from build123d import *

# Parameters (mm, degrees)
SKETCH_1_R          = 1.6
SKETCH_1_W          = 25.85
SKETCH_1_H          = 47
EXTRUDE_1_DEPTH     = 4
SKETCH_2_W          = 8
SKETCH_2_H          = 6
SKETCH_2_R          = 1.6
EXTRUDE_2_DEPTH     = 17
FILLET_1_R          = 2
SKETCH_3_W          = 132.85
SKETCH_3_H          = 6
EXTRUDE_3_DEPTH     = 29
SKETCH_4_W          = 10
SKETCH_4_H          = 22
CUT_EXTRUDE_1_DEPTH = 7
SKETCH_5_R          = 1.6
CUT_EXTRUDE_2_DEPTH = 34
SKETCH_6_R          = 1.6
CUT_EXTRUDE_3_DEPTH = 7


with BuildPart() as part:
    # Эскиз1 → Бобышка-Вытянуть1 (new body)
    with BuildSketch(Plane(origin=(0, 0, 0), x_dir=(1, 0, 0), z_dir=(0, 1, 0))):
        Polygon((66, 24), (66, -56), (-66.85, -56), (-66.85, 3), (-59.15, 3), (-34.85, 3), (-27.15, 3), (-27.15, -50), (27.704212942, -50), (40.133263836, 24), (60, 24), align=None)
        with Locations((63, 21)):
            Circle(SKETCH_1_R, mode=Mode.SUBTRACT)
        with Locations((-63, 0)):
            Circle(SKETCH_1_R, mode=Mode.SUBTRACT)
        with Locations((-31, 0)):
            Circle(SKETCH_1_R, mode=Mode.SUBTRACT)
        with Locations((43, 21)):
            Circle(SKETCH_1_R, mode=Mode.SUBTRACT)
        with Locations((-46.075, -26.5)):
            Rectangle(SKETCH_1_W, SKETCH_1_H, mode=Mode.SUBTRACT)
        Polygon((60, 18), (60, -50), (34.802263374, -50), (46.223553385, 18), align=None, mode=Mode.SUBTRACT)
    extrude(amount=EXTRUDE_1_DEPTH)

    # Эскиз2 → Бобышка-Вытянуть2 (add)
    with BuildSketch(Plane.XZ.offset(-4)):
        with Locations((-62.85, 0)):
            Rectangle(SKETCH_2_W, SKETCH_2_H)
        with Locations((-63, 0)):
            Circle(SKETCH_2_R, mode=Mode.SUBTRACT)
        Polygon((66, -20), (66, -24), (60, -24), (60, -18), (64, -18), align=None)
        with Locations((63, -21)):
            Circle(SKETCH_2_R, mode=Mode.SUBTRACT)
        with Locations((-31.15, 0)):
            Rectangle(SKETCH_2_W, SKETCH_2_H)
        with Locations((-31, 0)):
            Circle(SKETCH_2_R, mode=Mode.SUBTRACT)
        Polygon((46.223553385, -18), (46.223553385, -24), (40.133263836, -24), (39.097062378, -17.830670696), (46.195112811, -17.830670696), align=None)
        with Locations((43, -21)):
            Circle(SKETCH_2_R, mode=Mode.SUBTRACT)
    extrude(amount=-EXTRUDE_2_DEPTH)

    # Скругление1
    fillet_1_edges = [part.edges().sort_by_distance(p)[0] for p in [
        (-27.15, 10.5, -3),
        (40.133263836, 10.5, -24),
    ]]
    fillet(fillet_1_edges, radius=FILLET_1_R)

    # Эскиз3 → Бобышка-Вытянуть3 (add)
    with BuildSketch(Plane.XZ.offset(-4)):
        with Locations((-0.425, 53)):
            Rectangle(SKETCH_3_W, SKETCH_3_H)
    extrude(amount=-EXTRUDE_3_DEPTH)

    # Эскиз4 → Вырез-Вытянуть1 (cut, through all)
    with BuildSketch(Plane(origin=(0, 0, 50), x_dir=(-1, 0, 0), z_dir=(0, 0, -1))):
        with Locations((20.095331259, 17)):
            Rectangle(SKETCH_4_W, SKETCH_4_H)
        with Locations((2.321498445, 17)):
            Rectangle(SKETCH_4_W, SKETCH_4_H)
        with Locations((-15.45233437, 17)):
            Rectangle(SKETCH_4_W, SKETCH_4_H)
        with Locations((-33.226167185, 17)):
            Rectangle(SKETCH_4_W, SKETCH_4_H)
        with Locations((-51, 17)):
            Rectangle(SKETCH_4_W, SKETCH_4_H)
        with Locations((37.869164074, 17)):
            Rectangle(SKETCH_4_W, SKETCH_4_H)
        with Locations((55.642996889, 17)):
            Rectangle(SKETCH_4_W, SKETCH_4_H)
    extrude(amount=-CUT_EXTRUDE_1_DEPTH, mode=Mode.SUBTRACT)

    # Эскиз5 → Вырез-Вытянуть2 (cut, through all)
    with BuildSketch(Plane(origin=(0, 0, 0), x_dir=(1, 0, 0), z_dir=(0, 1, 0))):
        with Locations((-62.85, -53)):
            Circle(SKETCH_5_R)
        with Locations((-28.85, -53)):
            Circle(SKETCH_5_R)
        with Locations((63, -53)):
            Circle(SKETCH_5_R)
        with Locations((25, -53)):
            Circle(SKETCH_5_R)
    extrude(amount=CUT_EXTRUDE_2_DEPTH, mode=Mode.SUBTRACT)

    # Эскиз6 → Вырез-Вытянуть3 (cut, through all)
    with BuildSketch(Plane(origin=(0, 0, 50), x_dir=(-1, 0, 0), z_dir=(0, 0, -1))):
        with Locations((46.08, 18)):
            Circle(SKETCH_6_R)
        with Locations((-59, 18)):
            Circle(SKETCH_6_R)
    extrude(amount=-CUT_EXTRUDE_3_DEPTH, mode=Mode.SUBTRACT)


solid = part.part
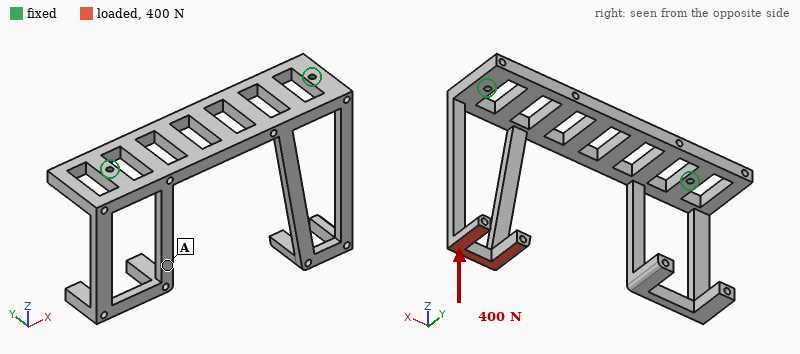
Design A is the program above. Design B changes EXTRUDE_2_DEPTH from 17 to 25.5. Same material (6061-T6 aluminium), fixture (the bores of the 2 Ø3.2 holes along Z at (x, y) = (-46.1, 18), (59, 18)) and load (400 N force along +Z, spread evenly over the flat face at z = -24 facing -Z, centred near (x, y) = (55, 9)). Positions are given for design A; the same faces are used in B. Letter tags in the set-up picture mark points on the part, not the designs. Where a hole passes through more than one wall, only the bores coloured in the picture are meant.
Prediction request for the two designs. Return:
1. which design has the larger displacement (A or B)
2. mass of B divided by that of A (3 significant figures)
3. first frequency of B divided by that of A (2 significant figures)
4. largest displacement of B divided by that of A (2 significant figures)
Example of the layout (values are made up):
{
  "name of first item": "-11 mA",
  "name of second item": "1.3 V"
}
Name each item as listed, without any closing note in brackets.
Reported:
{
  "which design has the larger displacement": "B",
  "mass of B divided by that of A": "1.05",
  "first frequency of B divided by that of A": "0.90",
  "largest displacement of B divided by that of A": "1.8"
}
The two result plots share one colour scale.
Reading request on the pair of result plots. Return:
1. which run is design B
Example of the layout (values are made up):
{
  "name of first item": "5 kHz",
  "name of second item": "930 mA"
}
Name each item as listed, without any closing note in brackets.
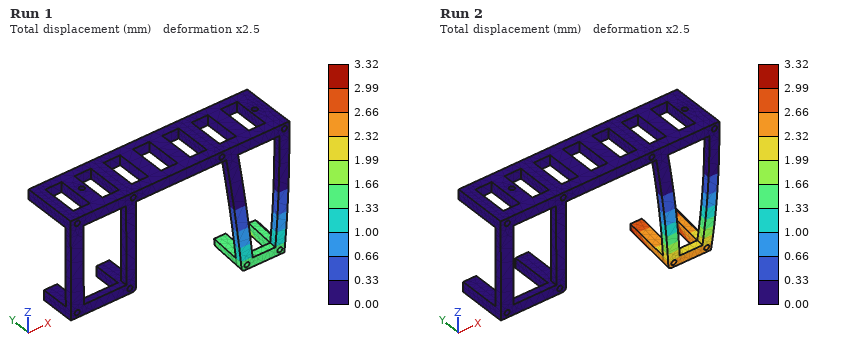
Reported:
{
  "which run is design B": "Run 2"
}
